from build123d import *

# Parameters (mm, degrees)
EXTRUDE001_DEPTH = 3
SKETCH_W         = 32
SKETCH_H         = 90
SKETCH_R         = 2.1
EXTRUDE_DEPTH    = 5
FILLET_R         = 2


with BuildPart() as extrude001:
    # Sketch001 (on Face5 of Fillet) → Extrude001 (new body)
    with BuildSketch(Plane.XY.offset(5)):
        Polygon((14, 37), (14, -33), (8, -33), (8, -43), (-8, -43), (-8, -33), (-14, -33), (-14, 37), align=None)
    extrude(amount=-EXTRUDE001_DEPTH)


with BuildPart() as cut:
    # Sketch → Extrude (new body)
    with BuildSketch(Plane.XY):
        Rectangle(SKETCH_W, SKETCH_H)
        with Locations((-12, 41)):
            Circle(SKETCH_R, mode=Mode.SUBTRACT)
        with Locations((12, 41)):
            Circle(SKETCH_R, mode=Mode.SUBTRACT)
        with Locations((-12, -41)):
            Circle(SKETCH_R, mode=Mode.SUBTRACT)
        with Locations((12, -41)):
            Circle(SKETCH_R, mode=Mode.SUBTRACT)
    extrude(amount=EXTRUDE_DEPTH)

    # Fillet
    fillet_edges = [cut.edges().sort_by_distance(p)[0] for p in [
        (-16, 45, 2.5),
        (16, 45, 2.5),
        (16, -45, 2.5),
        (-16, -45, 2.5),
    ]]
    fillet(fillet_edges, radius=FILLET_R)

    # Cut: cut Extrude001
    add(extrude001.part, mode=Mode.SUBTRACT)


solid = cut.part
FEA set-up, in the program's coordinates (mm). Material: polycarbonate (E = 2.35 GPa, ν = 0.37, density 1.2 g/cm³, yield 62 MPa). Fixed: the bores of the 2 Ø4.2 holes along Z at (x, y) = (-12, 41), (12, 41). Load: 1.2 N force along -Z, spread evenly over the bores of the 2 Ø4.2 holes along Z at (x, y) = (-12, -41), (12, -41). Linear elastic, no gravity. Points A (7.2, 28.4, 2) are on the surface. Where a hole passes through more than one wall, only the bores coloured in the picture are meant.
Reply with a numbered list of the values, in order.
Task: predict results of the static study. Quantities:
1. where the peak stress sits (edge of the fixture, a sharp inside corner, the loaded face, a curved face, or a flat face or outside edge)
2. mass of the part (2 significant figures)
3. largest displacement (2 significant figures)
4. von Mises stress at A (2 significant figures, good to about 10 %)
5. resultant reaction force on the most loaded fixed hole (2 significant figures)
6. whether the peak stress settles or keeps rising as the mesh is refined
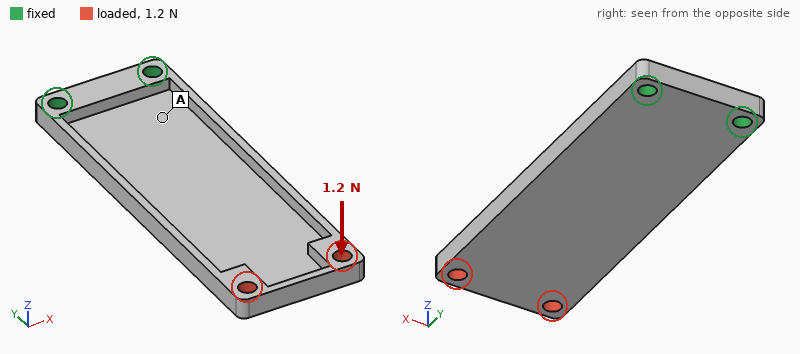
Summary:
1. a sharp inside corner
2. 9.3 g
3. 1.0 mm
4. 0.60 MPa
5. 3.0 N
6. keeps rising
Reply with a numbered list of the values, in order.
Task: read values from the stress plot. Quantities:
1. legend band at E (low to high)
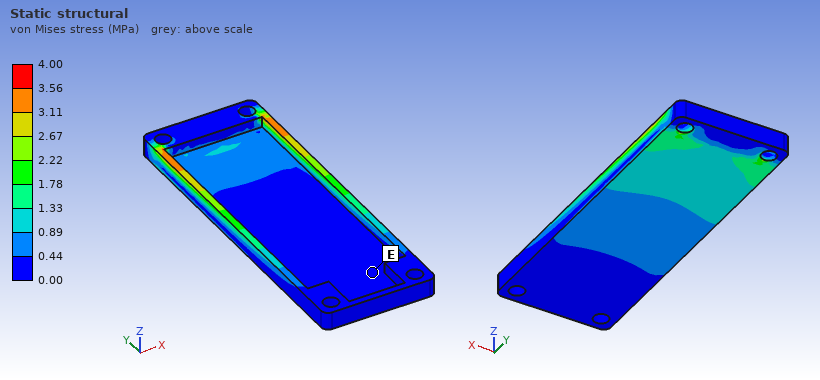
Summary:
1. 0.00 to 0.44 MPa
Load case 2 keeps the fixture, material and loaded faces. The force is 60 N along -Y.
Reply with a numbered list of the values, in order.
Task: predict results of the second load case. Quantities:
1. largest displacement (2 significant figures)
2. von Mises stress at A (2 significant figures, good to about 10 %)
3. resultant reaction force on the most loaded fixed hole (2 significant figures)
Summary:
1. 1.0 mm
2. 1.2 MPa
3. 30 N
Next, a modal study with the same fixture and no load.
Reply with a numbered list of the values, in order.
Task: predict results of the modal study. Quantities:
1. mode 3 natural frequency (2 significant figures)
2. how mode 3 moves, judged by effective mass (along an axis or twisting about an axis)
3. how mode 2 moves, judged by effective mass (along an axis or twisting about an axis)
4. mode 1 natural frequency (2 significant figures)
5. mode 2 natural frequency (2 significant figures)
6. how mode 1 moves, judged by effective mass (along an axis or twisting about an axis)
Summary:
1. 700 Hz
2. along Z
3. twisting about Y
4. 110 Hz
5. 350 Hz
6. along Z
